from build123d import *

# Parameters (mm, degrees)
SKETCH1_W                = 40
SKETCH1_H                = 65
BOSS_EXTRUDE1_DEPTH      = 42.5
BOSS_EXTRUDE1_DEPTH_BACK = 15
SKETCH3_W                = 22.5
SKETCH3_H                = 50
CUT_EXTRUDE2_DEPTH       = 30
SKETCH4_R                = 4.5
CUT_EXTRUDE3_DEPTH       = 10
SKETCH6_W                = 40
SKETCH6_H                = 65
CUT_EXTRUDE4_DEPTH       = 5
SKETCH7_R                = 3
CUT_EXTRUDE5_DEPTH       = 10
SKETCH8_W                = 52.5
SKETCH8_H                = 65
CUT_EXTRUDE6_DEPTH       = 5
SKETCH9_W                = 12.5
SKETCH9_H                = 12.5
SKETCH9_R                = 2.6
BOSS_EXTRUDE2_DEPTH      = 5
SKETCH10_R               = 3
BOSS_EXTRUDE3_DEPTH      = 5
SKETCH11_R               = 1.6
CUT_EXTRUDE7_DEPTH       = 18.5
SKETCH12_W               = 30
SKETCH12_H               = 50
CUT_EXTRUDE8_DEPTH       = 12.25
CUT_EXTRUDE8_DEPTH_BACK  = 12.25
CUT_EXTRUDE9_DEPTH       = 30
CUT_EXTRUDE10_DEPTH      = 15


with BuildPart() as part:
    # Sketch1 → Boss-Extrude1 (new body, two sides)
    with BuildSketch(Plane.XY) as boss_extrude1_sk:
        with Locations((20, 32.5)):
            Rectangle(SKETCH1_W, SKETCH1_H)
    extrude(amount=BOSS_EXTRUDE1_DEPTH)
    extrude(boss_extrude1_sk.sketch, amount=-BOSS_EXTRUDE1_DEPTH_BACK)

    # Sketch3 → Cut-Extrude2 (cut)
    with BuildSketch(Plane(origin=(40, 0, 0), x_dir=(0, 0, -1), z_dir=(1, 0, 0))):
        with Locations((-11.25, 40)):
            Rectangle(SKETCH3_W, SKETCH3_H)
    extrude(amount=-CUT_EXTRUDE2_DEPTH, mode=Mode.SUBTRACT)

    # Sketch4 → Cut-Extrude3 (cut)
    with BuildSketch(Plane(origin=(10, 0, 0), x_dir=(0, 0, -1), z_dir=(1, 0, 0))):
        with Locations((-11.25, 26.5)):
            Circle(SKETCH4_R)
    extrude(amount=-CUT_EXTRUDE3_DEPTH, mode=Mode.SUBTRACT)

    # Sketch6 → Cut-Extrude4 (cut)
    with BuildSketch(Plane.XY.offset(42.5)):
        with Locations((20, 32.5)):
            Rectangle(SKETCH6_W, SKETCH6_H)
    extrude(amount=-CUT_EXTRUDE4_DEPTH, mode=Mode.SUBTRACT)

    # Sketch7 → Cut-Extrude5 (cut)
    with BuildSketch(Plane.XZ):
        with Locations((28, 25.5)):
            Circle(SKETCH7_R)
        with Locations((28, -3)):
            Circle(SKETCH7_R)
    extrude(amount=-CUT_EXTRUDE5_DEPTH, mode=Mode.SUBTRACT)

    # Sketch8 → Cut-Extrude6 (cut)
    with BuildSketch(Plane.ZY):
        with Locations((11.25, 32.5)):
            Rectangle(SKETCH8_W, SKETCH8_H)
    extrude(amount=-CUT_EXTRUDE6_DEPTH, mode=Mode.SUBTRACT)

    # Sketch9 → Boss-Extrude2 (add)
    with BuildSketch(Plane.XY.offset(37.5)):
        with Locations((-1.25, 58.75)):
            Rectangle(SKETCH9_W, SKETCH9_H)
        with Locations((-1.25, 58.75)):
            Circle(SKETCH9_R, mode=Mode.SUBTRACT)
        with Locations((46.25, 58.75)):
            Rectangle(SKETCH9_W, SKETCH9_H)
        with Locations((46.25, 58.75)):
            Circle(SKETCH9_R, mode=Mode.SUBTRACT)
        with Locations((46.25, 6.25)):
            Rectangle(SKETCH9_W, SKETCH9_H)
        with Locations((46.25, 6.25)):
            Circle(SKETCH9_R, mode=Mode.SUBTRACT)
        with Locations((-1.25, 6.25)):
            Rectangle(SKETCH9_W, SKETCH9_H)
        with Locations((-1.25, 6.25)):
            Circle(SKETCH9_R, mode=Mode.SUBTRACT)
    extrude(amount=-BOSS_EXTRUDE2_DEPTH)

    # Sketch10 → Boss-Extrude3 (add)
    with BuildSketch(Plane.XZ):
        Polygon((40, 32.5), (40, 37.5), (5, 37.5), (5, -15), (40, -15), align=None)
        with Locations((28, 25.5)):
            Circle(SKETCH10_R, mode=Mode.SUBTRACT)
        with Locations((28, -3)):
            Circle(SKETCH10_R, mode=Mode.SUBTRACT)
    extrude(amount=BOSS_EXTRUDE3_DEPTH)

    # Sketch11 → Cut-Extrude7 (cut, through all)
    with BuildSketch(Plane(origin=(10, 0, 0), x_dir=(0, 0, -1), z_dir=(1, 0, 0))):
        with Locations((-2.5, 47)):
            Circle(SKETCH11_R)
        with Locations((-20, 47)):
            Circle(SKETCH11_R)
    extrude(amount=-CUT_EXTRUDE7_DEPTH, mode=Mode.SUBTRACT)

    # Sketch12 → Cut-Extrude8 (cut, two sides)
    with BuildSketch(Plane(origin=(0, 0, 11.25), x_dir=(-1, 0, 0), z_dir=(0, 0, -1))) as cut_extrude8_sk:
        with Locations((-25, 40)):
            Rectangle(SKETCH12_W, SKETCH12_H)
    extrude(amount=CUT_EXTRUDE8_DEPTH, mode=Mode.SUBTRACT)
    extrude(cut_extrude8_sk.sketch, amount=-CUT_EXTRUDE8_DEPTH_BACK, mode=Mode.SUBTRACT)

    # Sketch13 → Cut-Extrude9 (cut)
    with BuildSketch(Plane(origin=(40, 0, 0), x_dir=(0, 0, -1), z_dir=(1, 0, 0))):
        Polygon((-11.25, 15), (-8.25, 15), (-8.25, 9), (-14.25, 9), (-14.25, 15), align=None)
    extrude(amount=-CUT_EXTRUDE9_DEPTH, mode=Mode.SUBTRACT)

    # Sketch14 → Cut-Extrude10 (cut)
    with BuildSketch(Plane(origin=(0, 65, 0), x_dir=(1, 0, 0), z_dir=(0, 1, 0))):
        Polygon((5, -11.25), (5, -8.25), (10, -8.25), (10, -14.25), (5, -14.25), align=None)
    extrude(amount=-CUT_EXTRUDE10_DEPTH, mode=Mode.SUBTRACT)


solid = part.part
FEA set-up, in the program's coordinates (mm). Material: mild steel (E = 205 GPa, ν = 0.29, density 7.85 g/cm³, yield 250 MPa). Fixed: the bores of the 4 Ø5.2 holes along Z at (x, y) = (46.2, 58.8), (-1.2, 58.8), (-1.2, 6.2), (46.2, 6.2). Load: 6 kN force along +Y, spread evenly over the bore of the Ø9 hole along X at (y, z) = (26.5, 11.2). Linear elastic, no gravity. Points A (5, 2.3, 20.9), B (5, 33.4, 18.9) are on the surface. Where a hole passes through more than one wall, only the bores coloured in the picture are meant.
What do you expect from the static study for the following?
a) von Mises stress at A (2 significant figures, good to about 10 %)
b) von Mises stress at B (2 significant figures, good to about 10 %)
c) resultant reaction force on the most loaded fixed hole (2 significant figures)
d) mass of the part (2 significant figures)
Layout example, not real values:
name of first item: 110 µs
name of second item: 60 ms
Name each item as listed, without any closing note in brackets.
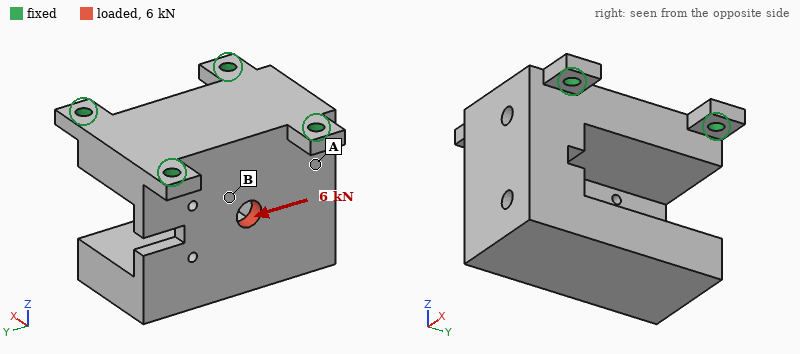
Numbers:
von Mises stress at A: 17 MPa
von Mises stress at B: 41 MPa
resultant reaction force on the most loaded fixed hole: 2.5 kN
mass of the part: 720 g
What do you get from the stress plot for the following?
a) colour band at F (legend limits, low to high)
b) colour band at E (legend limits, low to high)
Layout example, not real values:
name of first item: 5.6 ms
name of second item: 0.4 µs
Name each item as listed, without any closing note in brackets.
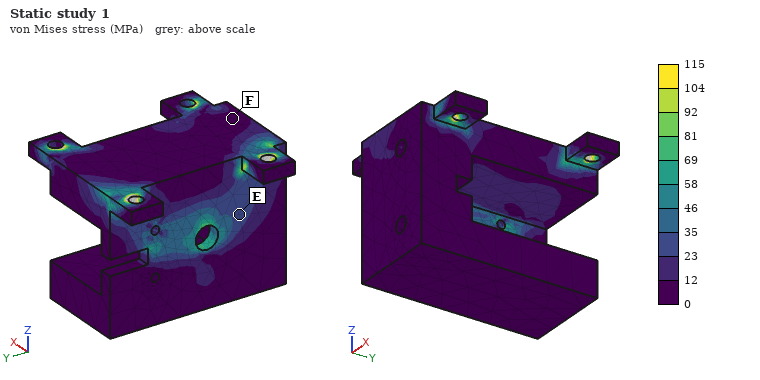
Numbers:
colour band at F: 0 to 12 MPa
colour band at E: 23 to 35 MPa
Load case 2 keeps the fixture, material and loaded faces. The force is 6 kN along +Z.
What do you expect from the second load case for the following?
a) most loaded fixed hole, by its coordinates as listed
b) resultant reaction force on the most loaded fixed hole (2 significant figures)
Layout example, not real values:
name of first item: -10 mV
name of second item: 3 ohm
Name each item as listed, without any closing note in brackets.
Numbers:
most loaded fixed hole, by its coordinates as listed: (-1.2, 6.2)
resultant reaction force on the most loaded fixed hole: 3.3 kN
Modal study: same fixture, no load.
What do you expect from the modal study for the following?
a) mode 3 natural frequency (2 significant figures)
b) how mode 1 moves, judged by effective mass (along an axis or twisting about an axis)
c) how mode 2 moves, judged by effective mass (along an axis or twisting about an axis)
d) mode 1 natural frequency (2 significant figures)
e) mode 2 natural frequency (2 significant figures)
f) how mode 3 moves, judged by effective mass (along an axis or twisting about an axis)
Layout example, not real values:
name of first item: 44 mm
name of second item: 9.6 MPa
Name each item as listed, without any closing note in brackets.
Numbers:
mode 3 natural frequency: 5000 Hz
how mode 1 moves, judged by effective mass: along X
how mode 2 moves, judged by effective mass: along Y
mode 1 natural frequency: 2500 Hz
mode 2 natural frequency: 3000 Hz
how mode 3 moves, judged by effective mass: along Z
